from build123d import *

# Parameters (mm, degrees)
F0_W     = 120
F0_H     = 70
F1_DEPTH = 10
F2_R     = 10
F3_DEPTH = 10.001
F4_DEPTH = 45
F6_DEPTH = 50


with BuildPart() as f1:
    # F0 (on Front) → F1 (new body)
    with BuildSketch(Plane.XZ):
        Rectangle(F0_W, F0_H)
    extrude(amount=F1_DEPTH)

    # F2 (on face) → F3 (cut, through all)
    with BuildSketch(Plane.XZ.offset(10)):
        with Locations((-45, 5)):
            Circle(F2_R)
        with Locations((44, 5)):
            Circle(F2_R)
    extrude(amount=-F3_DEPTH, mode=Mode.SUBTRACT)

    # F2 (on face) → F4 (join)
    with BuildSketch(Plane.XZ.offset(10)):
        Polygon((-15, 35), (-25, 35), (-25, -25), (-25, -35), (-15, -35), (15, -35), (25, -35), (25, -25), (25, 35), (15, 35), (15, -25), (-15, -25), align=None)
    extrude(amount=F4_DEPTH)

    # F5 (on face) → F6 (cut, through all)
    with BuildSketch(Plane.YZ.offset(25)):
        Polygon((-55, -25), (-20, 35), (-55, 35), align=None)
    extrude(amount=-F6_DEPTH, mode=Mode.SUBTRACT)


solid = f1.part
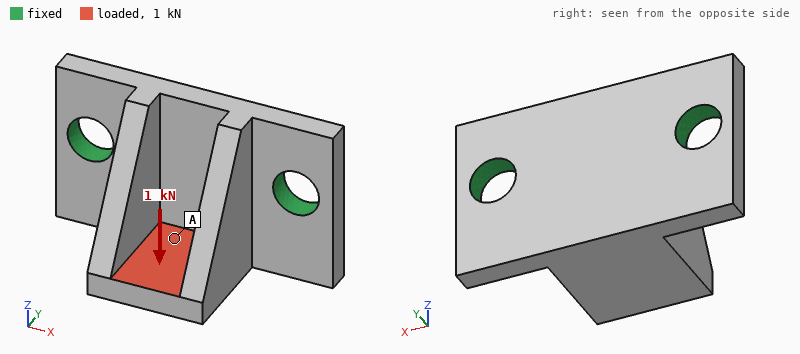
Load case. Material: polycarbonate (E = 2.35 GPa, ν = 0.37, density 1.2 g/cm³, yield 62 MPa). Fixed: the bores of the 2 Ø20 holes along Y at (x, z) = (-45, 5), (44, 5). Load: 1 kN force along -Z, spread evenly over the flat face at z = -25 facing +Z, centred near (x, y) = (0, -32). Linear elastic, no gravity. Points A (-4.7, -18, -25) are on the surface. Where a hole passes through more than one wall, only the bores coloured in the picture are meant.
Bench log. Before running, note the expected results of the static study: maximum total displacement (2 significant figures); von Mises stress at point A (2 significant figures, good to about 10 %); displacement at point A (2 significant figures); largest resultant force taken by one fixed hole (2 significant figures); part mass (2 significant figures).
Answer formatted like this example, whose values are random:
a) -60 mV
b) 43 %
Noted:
a) 0.67 mm
b) 1.8 MPa
c) 0.30 mm
d) 510 N
e) 160 g
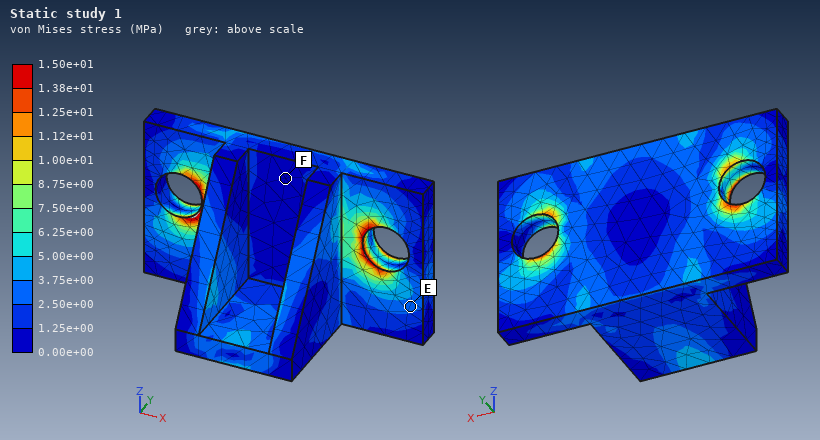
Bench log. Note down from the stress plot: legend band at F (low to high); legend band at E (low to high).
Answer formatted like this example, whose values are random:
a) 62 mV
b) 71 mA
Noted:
a) 0.00e+00 to 1.25e+00 MPa
b) 2.50e+00 to 3.75e+00 MPa
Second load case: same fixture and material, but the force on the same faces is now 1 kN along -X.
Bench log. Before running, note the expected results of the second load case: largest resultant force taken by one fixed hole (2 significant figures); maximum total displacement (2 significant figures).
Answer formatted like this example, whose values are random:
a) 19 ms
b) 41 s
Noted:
a) 710 N
b) 0.37 mm
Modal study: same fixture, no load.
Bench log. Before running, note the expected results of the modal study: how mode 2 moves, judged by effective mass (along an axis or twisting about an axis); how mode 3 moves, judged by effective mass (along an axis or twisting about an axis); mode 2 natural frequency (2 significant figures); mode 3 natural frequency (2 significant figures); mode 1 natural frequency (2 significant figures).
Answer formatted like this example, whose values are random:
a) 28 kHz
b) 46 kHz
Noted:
a) along X
b) along Y
c) 1400 Hz
d) 1700 Hz
e) 830 Hz
